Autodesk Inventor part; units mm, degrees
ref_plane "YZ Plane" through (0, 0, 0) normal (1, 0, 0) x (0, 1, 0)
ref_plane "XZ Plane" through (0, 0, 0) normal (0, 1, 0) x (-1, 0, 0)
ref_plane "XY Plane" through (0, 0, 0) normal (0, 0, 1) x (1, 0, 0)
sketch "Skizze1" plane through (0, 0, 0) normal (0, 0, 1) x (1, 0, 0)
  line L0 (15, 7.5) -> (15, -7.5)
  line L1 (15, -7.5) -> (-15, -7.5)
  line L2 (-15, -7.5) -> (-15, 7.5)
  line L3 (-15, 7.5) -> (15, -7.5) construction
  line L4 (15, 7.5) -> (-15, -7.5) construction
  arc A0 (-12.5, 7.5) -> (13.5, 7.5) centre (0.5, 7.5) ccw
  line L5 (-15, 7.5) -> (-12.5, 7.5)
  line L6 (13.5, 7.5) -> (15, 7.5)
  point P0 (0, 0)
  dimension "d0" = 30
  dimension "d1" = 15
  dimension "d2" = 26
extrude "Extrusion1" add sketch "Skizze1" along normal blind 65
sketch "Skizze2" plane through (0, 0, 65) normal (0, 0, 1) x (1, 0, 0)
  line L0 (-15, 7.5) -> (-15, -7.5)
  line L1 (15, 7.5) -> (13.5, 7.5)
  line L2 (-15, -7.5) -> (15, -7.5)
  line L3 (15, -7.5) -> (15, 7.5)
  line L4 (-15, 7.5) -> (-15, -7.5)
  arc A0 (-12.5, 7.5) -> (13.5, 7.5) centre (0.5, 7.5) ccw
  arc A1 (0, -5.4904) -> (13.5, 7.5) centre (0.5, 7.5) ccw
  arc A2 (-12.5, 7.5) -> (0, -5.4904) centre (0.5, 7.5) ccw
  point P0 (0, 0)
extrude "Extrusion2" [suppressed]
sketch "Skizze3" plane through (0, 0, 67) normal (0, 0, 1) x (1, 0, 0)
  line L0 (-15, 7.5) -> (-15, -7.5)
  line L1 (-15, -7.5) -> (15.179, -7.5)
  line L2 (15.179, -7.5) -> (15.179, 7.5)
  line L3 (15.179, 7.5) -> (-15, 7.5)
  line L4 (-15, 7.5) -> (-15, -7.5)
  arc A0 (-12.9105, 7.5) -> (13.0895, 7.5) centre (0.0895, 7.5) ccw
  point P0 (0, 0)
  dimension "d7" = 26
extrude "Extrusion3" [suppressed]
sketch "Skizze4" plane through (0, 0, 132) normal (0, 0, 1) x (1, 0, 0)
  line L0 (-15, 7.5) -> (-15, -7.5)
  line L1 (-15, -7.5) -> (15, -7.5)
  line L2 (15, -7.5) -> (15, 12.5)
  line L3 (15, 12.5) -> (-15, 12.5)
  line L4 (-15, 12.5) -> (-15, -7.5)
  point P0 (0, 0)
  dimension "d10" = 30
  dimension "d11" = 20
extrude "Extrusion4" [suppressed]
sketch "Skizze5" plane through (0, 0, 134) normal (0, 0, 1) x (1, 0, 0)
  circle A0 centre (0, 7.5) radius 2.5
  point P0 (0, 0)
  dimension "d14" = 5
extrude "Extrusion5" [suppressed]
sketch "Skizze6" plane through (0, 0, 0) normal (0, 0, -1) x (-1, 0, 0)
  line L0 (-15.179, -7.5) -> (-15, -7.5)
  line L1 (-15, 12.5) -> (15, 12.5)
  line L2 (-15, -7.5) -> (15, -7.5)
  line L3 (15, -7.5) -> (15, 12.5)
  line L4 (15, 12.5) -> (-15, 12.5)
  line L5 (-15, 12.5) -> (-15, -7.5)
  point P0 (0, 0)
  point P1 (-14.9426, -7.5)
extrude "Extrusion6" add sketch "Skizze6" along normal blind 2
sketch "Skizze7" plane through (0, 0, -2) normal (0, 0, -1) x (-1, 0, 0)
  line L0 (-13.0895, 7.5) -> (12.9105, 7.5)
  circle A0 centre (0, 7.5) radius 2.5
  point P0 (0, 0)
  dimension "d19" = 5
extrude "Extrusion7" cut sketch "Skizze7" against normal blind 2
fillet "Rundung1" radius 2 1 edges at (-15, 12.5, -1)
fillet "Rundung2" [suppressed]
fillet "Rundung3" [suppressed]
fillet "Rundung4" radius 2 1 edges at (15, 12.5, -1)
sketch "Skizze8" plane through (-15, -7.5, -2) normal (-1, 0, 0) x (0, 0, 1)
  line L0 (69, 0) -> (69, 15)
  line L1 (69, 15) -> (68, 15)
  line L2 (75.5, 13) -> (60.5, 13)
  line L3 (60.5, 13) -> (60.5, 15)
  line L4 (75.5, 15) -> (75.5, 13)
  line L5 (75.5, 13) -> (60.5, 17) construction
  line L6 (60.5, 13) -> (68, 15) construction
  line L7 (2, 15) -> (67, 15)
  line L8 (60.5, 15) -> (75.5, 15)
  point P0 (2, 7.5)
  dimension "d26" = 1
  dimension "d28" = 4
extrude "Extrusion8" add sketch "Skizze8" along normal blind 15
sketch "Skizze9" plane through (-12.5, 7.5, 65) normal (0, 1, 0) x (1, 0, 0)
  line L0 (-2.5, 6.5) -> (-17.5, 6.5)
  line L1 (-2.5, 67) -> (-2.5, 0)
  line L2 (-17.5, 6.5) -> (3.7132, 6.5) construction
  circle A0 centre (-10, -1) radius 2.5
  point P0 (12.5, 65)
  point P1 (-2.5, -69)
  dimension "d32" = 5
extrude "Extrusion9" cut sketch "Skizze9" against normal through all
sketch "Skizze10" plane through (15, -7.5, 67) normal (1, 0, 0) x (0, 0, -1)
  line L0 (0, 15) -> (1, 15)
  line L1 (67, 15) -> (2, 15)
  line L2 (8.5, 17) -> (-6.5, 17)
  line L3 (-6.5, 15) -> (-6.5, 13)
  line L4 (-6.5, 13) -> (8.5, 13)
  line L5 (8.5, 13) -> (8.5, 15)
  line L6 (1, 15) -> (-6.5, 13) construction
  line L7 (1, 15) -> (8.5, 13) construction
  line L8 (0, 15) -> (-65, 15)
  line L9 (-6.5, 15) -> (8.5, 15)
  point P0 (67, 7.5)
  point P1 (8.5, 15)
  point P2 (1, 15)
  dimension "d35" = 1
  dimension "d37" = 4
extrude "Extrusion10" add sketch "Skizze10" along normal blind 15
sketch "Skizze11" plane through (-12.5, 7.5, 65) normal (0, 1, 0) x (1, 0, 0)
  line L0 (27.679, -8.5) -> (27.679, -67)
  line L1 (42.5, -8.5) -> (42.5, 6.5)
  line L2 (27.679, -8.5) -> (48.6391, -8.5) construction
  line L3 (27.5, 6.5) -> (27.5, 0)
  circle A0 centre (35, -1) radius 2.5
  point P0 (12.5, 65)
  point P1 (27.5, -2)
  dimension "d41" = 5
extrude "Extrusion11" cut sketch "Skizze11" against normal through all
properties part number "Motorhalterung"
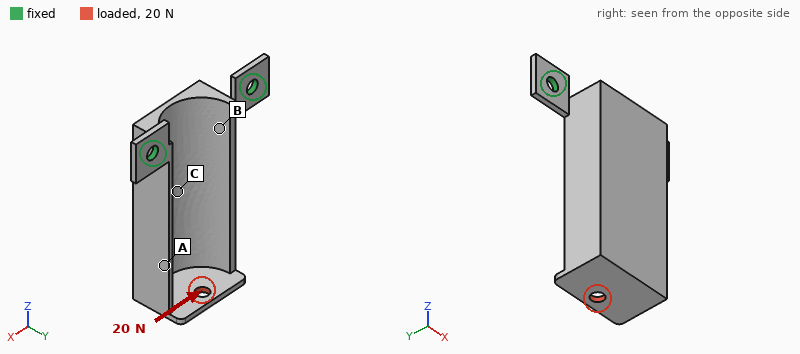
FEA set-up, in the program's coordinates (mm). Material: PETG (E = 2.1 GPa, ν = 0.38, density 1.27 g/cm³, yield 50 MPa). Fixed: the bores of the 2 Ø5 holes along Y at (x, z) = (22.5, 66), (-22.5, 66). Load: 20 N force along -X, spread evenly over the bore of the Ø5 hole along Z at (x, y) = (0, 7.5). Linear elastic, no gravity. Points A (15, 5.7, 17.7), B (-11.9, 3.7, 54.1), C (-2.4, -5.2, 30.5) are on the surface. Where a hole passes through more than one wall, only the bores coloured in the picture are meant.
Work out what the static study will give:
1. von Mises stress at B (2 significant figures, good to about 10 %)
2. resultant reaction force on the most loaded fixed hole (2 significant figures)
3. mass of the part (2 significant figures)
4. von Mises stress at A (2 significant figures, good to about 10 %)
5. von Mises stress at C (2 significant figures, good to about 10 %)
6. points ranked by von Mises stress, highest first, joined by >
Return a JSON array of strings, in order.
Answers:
["4.3 MPa", "40 N", "18 g", "1.1 MPa", "2.1 MPa", "B > C > A"]
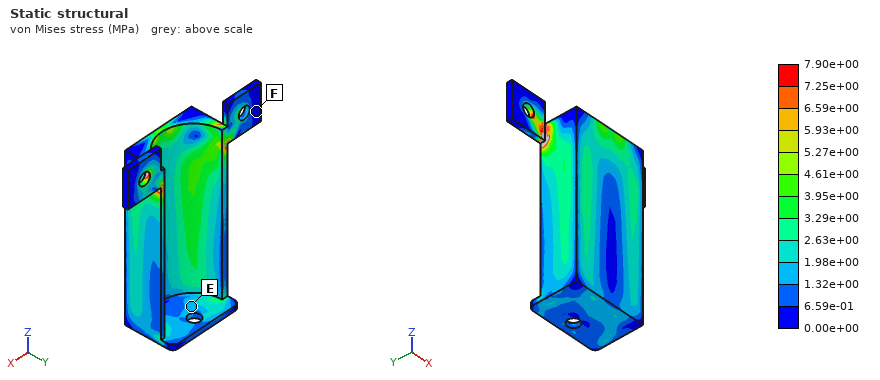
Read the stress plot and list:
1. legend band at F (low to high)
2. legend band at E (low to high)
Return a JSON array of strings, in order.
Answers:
["0.00e+00 to 6.59e-01 MPa", "1.32e+00 to 1.98e+00 MPa"]
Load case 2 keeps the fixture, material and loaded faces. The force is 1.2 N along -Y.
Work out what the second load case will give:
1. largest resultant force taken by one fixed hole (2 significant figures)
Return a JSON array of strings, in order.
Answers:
["0.92 N"]
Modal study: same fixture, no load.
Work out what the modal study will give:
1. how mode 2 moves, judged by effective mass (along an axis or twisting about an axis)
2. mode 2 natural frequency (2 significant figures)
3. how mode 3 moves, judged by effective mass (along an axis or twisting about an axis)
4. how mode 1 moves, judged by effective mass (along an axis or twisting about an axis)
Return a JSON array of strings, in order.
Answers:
["along X", "380 Hz", "along X", "along Y"]
